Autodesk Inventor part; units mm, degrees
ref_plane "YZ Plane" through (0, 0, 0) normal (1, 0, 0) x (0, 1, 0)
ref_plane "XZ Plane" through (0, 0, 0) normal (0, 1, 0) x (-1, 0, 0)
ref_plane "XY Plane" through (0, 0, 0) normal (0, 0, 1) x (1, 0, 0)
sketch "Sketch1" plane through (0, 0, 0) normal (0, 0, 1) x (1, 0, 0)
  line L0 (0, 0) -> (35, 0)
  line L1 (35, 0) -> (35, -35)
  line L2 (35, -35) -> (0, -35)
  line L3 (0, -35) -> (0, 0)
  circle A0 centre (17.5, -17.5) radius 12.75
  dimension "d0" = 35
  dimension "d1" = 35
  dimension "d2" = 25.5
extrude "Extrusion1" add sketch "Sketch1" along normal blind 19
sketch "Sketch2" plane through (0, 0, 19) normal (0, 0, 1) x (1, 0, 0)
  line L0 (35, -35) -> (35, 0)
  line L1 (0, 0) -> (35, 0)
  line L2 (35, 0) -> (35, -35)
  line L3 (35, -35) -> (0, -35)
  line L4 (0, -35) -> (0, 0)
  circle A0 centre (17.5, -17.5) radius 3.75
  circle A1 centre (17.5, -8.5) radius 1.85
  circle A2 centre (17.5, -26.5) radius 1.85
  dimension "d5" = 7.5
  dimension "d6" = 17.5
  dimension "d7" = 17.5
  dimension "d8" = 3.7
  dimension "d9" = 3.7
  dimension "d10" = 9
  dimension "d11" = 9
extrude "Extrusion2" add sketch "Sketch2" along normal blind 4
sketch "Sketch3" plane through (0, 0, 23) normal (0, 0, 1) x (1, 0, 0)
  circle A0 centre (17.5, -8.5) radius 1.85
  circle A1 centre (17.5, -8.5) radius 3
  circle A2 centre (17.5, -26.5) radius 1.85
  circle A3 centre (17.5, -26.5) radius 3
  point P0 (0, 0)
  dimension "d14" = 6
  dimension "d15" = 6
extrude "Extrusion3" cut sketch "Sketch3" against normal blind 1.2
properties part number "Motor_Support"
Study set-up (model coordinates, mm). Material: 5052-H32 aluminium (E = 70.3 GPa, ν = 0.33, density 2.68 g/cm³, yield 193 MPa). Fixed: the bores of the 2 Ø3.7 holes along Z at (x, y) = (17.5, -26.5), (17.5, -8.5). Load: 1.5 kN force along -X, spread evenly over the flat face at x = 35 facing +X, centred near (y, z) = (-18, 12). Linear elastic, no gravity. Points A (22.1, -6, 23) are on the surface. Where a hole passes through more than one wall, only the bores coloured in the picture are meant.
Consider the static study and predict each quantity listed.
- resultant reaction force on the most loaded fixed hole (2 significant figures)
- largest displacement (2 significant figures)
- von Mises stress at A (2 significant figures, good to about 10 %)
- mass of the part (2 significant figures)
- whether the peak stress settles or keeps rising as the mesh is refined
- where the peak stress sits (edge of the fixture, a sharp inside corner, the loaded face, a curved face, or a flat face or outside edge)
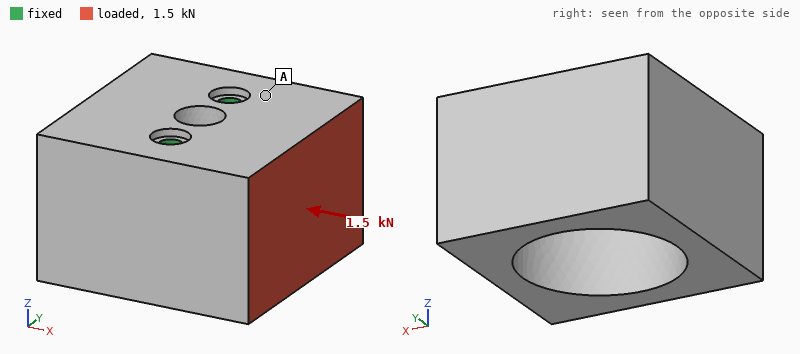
760 N
0.11 mm
24 MPa
49 g
keeps rising
edge of the fixture
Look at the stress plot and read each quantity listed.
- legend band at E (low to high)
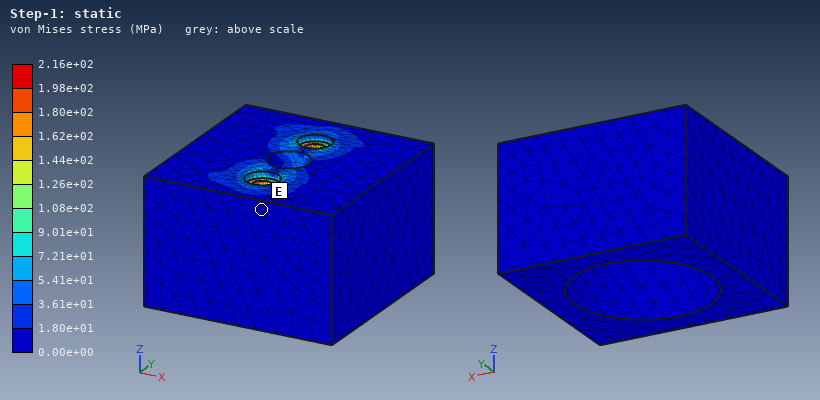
0.00e+00 to 1.80e+01 MPa
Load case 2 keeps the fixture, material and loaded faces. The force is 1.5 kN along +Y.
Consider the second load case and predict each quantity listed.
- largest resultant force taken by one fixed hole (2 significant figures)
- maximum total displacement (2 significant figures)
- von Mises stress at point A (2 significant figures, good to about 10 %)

1.6 kN
30 µm
22 MPa
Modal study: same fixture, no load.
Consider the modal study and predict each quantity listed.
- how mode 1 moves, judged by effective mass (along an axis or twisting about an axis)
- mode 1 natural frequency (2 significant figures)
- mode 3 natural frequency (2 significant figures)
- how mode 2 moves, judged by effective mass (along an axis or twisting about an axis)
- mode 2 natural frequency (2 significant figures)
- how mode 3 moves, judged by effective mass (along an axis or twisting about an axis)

along X
2700 Hz
11 kHz
along Y
7100 Hz
twisting about Z
